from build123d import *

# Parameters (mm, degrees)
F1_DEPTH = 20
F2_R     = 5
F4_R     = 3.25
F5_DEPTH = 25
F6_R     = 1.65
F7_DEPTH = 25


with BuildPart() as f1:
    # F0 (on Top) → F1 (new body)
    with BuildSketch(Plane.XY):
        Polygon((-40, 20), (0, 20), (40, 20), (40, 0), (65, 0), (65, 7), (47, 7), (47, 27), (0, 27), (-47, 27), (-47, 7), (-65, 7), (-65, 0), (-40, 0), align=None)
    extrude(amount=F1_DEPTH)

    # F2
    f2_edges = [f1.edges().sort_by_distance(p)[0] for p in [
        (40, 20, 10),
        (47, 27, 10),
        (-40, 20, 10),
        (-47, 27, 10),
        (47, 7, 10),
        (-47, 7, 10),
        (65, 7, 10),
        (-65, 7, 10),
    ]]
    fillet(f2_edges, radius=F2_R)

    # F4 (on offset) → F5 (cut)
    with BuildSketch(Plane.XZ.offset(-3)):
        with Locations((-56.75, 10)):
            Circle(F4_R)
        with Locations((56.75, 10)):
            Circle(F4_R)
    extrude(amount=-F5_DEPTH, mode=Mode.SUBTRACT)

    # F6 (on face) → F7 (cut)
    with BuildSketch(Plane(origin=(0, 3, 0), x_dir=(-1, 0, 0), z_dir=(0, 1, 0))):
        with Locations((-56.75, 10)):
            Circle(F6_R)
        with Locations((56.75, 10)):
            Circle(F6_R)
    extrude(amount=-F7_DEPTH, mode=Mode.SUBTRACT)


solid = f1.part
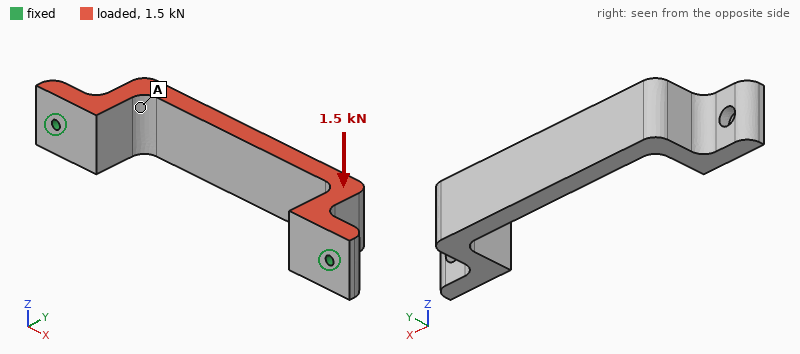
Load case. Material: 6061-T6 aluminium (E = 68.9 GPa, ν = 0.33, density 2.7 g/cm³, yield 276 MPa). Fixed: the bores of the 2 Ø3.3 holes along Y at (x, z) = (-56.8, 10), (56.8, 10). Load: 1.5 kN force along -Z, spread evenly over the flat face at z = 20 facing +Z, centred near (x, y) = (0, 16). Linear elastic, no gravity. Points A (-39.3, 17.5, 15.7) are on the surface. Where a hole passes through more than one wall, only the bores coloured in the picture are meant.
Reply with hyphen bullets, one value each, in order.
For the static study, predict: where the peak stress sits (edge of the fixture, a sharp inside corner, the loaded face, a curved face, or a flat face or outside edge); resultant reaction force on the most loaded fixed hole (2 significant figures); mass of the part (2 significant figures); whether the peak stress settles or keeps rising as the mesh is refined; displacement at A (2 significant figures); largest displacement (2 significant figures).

- edge of the fixture
- 750 N
- 63 g
- keeps rising
- 0.16 mm
- 0.26 mm
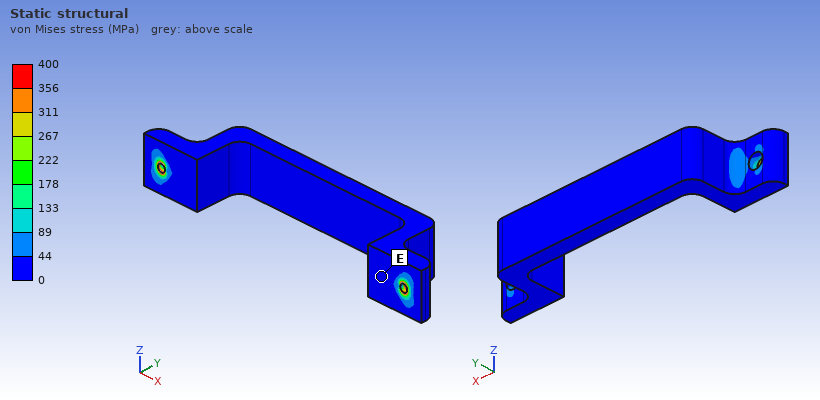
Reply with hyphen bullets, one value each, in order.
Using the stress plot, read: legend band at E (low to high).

- 0 to 44 MPa
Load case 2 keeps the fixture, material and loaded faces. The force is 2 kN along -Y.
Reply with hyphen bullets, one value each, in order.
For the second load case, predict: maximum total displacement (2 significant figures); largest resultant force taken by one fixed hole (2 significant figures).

- 0.23 mm
- 1.3 kN
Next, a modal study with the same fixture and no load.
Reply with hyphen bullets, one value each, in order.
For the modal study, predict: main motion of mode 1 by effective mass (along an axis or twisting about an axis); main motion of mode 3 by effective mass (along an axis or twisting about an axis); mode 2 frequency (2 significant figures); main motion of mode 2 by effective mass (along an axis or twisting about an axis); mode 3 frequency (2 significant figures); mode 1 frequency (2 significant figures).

- along Z
- twisting about Y
- 3200 Hz
- along X
- 4200 Hz
- 1700 Hz
